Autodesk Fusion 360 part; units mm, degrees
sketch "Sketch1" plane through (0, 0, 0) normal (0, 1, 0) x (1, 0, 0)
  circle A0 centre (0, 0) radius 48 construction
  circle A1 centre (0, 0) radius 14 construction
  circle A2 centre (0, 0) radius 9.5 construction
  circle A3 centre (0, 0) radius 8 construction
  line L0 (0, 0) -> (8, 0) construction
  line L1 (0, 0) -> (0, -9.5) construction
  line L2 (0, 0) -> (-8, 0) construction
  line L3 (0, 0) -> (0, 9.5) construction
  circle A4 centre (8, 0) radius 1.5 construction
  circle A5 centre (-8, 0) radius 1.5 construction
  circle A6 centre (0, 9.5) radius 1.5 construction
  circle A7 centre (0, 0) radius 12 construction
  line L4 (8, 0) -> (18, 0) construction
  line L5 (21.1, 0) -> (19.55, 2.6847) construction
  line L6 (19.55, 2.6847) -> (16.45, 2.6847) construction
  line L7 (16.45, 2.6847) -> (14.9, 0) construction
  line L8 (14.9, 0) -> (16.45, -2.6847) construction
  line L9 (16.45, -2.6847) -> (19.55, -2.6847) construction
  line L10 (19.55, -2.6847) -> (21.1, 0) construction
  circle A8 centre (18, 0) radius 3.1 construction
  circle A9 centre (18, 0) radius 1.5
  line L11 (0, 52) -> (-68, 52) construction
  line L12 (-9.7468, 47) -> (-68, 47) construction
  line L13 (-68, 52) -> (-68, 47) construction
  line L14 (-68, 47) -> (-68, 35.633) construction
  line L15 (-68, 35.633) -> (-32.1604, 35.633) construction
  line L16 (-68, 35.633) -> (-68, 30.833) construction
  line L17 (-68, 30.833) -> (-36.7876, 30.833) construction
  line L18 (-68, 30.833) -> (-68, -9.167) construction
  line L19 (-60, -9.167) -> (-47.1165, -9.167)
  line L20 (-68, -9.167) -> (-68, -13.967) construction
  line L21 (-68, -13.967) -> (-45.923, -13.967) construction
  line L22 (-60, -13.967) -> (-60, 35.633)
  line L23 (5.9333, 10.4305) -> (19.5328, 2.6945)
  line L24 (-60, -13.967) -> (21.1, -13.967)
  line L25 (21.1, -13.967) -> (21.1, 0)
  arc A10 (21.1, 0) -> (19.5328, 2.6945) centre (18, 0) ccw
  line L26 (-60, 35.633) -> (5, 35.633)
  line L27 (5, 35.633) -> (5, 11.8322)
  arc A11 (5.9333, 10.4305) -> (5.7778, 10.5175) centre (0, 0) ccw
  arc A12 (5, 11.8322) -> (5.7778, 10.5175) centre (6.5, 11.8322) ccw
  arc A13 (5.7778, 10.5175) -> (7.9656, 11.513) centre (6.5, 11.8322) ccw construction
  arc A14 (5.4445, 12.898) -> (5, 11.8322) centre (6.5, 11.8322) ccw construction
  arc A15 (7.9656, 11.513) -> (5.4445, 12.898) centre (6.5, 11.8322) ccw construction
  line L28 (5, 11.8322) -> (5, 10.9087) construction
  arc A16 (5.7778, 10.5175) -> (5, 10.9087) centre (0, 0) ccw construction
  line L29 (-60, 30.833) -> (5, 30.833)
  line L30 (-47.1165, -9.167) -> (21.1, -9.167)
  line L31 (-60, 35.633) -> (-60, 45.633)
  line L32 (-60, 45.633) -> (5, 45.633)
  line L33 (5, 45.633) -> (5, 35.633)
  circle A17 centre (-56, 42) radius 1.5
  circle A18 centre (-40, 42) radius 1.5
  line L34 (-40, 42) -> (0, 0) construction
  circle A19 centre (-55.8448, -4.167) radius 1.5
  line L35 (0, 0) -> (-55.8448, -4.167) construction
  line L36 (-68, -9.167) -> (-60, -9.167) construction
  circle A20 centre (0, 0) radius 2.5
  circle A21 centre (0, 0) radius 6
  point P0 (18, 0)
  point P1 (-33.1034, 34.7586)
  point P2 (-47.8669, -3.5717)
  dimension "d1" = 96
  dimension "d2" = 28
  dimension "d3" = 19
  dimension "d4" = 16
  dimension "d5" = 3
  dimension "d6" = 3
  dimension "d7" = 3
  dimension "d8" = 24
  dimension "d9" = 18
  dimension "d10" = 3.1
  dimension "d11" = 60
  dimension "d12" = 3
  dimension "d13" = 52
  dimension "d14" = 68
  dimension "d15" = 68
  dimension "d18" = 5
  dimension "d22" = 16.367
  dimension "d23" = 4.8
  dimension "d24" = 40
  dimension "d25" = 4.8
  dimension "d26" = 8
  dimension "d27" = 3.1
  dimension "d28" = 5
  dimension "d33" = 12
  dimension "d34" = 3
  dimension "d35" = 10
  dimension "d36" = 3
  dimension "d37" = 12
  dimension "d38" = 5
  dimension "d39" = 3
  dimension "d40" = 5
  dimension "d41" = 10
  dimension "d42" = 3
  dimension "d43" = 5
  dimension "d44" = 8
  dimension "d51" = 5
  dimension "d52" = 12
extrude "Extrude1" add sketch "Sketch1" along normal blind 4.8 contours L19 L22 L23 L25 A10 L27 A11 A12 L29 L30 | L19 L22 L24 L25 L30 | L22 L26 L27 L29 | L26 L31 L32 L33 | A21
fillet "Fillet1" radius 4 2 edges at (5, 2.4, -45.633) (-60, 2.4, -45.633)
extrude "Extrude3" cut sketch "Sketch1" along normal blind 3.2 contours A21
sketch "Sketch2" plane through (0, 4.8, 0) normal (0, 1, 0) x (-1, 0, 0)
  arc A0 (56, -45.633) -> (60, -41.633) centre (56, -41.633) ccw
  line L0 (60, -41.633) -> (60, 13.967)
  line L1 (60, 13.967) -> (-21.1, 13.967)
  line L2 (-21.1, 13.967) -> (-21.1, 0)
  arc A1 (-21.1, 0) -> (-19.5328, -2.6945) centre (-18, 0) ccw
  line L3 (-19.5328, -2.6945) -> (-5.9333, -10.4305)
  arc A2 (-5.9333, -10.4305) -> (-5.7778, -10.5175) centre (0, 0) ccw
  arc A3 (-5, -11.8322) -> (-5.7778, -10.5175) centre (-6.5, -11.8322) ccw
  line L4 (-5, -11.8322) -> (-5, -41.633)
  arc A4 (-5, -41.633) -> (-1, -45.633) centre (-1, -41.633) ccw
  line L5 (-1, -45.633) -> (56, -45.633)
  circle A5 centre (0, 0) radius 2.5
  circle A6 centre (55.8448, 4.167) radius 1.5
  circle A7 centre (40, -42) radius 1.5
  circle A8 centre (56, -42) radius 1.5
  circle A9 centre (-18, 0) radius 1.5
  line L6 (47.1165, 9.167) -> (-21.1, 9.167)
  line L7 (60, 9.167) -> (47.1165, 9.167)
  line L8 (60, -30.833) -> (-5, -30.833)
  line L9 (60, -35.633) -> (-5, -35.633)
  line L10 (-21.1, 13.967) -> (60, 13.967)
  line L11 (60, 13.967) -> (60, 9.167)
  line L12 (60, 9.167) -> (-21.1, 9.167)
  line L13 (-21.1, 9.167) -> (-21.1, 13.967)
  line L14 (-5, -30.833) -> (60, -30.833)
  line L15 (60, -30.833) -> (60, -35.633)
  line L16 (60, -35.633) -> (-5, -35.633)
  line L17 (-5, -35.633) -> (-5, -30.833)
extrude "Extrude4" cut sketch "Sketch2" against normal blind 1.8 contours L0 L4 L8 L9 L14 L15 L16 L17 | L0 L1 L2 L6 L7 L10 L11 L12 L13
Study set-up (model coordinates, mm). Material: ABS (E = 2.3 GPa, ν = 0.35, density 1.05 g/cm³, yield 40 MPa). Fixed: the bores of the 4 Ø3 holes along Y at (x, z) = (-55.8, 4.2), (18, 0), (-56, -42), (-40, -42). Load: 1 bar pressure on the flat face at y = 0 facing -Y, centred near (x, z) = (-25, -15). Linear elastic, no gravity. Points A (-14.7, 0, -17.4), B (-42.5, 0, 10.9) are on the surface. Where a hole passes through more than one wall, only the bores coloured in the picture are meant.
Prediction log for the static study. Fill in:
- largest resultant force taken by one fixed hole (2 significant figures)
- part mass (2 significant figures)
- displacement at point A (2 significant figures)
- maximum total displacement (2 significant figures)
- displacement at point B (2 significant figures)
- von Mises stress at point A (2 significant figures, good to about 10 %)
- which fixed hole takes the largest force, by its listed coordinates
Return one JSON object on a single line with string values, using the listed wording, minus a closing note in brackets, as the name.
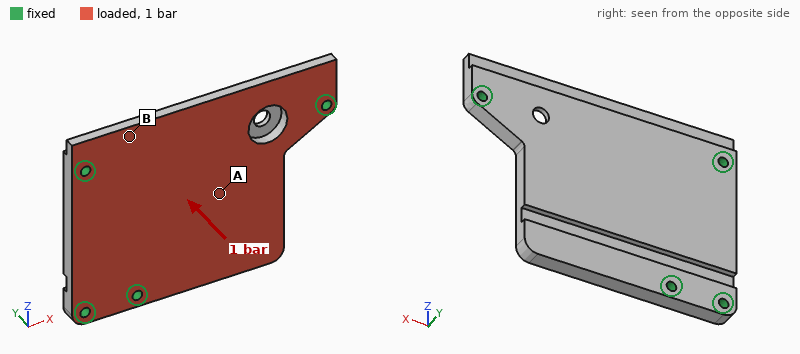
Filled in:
{"largest resultant force taken by one fixed hole": "170 N", "part mass": "19 g", "displacement at point A": "0.61 mm", "maximum total displacement": "1.2 mm", "displacement at point B": "0.21 mm", "von Mises stress at point A": "7.0 MPa", "which fixed hole takes the largest force, by its listed coordinates": "(-40, -42)"}
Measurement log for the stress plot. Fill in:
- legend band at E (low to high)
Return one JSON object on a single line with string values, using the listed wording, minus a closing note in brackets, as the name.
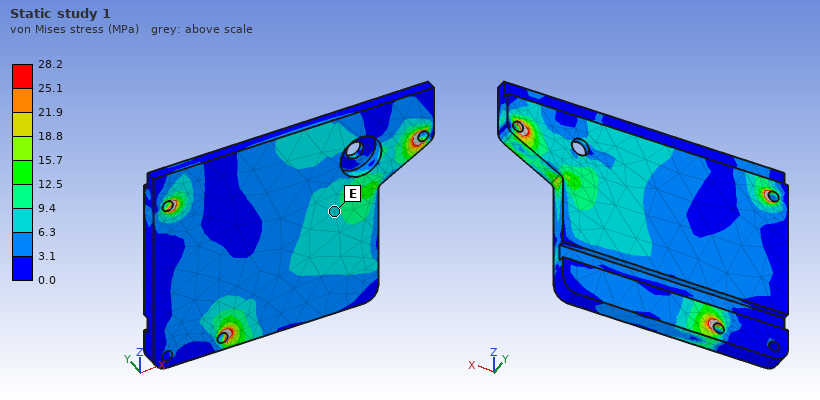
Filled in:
{"legend band at E": "6.3 to 9.4 MPa"}
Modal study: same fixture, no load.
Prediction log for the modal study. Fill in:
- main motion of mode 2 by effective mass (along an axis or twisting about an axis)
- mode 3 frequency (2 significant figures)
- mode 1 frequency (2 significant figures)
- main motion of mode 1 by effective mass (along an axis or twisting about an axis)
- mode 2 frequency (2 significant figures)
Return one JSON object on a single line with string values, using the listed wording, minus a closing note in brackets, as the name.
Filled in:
{"main motion of mode 2 by effective mass": "along Y", "mode 3 frequency": "2500 Hz", "mode 1 frequency": "890 Hz", "main motion of mode 1 by effective mass": "along Y", "mode 2 frequency": "1200 Hz"}
